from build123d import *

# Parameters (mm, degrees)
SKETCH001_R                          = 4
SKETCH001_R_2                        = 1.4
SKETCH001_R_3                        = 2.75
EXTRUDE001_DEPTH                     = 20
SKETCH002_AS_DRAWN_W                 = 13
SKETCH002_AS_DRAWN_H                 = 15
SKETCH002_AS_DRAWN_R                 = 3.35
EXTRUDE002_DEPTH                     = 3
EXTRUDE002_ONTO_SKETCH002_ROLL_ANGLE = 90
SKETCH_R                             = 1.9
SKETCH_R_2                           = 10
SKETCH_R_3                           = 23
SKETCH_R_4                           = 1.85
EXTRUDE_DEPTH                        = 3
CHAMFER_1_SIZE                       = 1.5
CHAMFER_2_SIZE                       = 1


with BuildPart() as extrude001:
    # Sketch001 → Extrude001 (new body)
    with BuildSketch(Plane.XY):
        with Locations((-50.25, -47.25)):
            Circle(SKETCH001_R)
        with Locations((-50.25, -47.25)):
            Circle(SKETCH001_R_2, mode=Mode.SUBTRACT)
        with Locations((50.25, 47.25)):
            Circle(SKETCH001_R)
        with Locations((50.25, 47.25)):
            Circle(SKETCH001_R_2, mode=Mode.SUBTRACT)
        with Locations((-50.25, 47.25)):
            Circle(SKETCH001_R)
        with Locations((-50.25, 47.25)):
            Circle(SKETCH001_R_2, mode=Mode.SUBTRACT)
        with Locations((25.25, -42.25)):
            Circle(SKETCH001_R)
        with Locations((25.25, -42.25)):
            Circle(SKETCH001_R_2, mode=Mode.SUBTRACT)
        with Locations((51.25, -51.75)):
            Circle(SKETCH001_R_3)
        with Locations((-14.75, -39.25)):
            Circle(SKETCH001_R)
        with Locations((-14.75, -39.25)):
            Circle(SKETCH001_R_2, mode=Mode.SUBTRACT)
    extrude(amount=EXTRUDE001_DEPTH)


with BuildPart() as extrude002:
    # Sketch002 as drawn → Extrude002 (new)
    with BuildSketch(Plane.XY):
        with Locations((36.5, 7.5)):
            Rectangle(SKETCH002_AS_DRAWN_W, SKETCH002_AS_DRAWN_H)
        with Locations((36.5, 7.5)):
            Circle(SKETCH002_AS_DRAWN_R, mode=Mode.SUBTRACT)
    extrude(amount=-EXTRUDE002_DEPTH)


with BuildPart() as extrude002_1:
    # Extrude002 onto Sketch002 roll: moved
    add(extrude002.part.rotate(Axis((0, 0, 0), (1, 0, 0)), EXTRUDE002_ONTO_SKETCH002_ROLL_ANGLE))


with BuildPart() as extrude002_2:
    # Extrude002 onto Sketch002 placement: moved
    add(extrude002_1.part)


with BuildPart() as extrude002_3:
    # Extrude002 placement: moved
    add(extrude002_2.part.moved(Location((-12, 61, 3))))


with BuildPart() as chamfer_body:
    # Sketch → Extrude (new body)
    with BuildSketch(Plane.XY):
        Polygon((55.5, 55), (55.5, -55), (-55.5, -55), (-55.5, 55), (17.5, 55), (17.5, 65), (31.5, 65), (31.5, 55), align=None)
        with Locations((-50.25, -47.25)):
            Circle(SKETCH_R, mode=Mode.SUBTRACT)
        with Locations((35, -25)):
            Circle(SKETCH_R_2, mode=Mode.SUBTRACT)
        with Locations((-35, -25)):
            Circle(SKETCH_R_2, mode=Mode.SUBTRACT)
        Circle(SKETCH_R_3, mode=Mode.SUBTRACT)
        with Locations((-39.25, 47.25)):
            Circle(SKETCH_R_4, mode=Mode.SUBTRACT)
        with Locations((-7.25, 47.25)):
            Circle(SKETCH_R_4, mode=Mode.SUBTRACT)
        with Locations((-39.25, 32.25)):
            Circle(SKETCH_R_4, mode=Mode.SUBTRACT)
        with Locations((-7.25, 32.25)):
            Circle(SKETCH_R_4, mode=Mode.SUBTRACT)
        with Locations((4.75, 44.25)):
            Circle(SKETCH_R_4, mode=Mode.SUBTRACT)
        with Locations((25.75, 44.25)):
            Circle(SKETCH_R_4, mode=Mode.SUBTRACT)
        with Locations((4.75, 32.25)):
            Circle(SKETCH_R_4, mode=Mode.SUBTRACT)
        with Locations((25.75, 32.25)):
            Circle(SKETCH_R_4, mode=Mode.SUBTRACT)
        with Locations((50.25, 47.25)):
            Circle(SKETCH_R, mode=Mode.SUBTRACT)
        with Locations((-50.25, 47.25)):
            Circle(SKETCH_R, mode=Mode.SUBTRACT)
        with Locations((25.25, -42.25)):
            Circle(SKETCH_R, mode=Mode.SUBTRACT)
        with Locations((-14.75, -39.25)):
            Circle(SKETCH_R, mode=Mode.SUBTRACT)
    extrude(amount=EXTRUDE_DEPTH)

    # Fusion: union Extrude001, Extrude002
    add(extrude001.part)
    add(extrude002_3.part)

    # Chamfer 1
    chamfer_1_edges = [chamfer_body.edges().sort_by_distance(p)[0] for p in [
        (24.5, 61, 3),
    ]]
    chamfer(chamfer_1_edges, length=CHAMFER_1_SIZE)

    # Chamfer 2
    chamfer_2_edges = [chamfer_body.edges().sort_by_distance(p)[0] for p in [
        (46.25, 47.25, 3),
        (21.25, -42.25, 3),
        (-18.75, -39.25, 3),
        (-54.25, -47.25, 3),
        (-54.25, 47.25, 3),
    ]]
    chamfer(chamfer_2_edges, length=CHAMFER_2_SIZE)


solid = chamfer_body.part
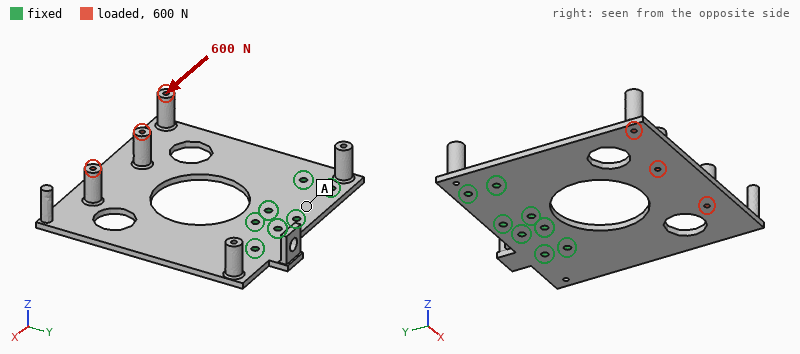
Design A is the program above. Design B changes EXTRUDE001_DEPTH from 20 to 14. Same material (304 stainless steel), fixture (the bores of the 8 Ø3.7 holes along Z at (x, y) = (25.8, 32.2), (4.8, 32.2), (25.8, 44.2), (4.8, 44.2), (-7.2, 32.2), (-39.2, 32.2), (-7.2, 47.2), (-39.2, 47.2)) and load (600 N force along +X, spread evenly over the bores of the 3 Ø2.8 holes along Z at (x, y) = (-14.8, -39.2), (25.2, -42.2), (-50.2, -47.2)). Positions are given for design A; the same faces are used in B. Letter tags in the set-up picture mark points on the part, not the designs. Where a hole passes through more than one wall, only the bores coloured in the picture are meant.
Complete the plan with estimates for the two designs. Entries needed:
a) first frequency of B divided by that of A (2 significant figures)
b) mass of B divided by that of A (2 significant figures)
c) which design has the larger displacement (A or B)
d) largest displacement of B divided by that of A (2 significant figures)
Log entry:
1.0
0.96
A
0.62
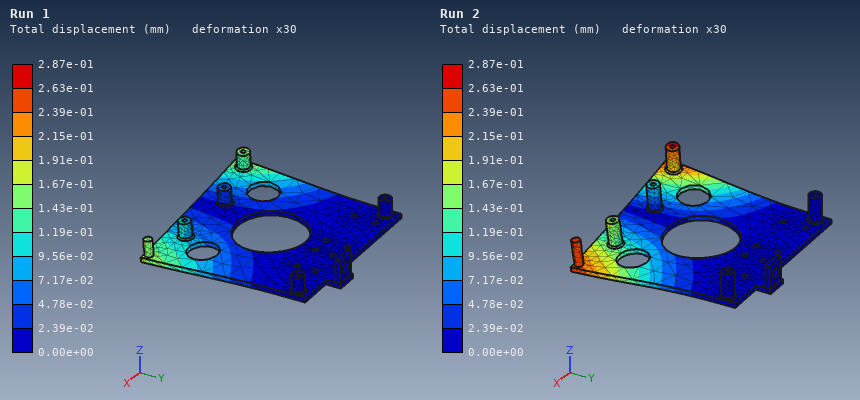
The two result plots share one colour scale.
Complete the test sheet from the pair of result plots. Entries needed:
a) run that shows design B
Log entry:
Run 1
